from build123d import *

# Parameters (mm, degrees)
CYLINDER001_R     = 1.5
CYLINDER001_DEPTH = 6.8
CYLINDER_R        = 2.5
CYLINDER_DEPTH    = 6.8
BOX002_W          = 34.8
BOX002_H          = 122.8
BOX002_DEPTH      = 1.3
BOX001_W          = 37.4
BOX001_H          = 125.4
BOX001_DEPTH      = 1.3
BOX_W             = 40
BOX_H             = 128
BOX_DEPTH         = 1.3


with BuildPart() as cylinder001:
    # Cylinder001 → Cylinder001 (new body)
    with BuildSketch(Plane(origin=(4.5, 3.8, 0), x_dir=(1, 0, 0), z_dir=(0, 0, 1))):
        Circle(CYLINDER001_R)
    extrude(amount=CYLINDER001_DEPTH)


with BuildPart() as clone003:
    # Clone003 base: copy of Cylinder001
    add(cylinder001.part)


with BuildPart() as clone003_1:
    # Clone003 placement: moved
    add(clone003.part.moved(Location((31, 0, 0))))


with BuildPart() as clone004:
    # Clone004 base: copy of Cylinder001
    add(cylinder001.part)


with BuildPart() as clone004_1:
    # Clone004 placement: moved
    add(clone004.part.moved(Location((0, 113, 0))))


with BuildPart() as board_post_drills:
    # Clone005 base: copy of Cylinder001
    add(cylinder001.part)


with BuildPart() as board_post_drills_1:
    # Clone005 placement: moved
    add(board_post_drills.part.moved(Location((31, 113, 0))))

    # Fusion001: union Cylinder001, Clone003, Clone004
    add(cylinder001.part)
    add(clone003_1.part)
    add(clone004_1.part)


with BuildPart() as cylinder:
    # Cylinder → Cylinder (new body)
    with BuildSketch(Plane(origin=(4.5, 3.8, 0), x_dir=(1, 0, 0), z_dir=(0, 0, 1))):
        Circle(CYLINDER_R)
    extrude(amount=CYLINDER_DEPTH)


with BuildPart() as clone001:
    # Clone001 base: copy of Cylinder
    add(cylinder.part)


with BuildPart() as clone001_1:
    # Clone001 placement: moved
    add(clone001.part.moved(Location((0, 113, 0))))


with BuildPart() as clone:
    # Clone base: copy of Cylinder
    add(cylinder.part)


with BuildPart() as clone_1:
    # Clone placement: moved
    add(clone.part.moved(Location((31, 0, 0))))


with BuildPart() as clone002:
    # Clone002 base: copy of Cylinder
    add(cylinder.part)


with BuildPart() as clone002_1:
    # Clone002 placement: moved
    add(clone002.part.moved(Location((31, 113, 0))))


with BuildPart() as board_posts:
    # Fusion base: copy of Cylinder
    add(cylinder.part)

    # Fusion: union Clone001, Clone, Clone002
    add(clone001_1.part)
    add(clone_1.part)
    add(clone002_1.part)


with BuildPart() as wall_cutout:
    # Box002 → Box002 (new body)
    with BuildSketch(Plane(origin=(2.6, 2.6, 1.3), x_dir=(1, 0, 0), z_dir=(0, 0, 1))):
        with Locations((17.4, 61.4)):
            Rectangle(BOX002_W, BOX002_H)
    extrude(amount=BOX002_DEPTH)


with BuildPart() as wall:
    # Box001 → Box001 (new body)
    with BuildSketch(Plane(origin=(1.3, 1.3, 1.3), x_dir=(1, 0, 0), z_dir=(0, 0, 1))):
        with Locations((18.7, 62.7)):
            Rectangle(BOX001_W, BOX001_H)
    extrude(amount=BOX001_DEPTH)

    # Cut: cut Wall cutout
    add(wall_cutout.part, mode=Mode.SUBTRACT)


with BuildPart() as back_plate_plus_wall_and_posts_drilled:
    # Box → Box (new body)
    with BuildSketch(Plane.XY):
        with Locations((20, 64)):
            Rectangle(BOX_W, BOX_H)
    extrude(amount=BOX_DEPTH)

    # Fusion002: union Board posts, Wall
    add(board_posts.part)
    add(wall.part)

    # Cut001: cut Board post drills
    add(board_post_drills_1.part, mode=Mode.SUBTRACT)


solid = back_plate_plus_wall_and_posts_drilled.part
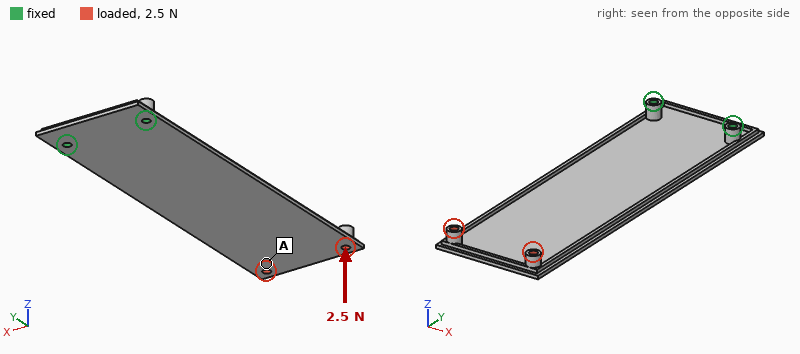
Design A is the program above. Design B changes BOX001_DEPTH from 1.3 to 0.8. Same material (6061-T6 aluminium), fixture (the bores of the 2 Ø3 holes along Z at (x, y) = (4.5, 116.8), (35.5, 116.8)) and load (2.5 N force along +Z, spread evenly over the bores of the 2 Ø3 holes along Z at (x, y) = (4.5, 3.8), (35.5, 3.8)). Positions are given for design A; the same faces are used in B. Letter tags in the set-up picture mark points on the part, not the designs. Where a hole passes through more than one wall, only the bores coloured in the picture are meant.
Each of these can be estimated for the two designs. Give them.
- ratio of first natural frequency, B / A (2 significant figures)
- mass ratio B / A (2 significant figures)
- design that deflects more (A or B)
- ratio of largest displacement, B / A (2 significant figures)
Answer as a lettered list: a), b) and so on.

a) 0.87
b) 0.97
c) B
d) 1.4
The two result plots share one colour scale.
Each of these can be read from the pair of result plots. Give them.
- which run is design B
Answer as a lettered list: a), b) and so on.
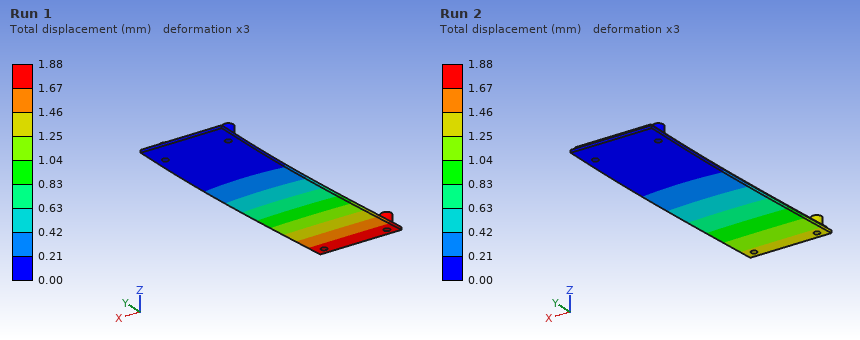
a) Run 1
